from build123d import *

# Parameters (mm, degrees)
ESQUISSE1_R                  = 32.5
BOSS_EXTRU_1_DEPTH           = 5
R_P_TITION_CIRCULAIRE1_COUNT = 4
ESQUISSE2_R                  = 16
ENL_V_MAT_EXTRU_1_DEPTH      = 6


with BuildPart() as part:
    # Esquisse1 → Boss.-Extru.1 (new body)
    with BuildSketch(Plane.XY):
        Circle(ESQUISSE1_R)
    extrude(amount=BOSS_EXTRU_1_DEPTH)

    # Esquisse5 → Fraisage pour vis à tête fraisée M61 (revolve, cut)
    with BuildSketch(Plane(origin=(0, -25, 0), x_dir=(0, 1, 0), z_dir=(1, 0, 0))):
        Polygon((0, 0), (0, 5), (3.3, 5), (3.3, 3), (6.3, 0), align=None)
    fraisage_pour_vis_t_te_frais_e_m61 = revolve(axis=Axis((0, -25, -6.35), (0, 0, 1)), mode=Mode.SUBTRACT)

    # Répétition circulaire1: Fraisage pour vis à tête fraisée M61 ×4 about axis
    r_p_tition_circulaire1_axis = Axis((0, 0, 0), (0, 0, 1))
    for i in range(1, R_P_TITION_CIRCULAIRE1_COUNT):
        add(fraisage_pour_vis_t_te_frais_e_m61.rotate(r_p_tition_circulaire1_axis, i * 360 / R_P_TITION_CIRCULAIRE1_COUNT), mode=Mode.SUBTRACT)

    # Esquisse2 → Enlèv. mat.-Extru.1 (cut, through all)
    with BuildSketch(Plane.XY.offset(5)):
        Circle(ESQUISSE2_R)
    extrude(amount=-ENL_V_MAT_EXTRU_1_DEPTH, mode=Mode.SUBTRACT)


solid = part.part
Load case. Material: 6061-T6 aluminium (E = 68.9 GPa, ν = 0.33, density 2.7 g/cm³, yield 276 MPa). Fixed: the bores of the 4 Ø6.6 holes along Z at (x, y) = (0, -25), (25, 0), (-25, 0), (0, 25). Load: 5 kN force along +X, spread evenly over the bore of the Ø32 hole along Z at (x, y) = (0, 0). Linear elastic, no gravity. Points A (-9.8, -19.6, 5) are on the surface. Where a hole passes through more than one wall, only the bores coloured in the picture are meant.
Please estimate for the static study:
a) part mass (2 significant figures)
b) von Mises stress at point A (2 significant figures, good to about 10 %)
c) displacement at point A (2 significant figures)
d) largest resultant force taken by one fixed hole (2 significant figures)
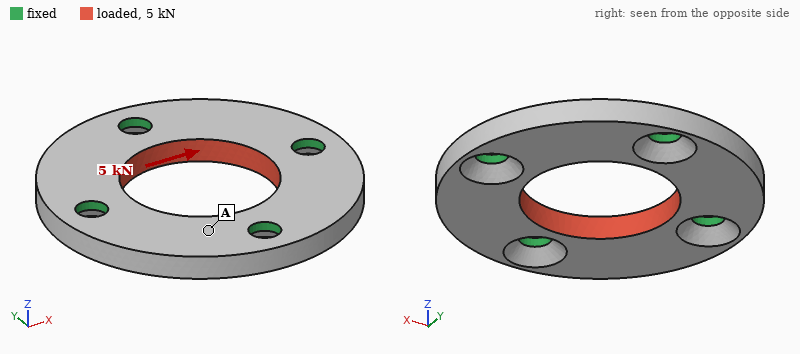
31 g
13 MPa
3.4 µm
1.3 kN
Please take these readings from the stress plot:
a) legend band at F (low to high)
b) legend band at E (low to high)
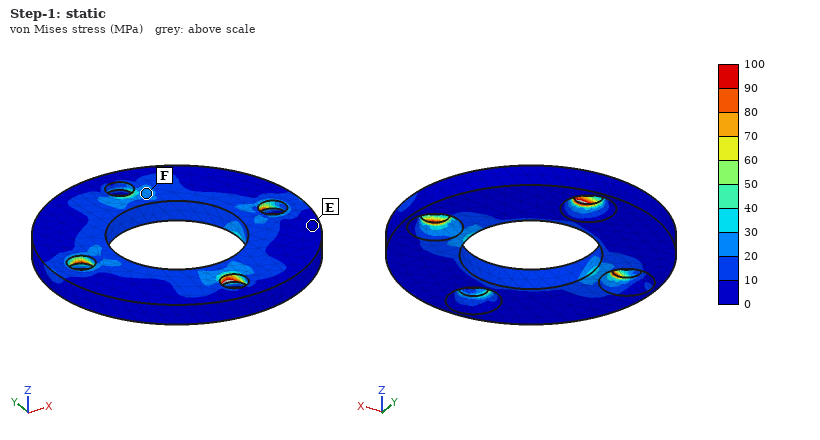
20 to 30 MPa
0 to 10 MPa
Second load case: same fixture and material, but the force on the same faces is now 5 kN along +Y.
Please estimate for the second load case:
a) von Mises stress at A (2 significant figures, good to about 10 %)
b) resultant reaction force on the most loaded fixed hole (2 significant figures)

12 MPa
1.3 kN
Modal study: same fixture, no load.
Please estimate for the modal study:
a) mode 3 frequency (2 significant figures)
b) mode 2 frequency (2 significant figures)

11 kHz
11 kHz
